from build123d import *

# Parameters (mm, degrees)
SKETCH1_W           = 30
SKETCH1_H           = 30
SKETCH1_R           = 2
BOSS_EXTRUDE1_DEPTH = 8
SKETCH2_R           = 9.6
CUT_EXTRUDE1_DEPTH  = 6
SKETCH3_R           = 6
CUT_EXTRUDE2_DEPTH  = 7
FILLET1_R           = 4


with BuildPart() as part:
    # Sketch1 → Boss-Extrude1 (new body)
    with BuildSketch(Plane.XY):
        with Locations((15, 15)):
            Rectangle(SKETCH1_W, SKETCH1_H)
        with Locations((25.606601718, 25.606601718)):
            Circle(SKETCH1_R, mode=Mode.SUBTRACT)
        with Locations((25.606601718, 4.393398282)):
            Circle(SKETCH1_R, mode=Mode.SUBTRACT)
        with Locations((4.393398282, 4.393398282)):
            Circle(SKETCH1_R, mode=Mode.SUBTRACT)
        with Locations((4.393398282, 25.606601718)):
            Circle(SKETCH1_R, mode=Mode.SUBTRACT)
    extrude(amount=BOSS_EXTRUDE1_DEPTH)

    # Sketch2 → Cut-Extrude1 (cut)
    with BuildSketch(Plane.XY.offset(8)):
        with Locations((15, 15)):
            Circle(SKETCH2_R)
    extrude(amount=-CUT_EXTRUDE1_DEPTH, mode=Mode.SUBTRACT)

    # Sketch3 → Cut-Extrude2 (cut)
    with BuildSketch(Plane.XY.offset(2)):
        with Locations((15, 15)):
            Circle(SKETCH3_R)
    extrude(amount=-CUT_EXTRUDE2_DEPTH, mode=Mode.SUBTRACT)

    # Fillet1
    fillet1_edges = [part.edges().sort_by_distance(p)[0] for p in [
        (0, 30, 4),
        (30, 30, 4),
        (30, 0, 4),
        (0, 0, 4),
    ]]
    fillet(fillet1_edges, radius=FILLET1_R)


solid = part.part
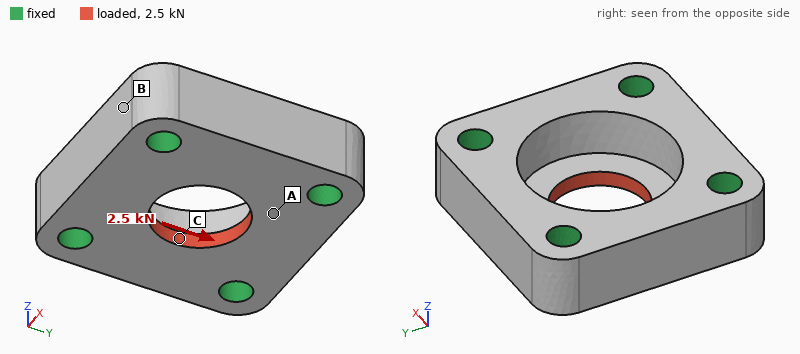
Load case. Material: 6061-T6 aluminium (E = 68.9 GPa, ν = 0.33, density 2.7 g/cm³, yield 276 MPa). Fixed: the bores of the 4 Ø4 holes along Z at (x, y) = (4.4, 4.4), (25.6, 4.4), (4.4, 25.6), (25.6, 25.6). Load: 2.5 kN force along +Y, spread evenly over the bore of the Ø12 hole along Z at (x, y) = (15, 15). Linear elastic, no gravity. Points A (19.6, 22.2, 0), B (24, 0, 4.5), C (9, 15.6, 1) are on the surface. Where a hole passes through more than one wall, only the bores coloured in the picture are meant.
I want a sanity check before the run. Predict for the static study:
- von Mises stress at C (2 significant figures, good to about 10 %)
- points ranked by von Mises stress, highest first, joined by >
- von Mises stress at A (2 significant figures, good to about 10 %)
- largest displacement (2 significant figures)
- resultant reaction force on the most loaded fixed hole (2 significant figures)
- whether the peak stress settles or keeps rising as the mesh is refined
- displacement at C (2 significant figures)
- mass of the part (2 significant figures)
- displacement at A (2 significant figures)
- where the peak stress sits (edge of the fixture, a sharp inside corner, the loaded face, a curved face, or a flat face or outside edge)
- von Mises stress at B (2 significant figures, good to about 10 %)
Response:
57 MPa
C > A > B
31 MPa
6.8 µm
650 N
keeps rising
4.1 µm
13 g
3.7 µm
edge of the fixture
11 MPa
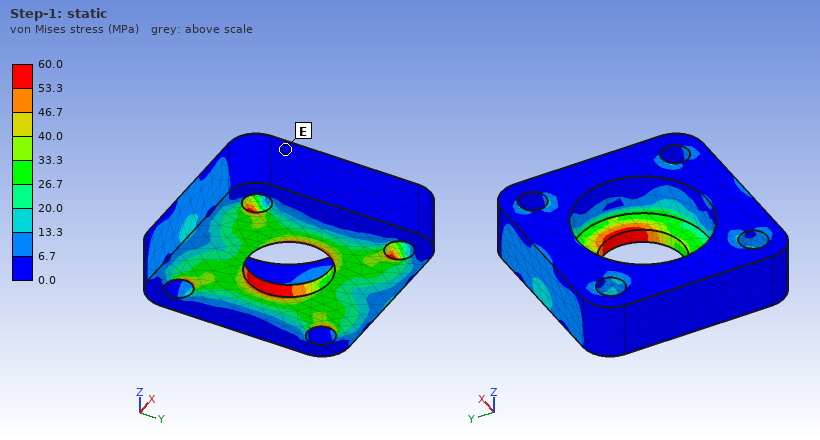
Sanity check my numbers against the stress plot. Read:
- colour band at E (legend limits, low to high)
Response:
0.0 to 6.7 MPa
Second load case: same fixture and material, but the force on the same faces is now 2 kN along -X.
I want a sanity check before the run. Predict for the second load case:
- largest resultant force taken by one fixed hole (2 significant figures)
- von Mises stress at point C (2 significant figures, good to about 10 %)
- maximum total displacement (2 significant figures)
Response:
520 N
25 MPa
5.4 µm
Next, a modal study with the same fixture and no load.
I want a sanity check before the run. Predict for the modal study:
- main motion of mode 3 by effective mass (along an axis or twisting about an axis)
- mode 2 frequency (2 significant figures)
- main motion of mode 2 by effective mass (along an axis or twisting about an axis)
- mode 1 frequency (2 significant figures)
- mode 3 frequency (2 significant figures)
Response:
twisting about Y
62 kHz
along Z
56 kHz
65 kHz
